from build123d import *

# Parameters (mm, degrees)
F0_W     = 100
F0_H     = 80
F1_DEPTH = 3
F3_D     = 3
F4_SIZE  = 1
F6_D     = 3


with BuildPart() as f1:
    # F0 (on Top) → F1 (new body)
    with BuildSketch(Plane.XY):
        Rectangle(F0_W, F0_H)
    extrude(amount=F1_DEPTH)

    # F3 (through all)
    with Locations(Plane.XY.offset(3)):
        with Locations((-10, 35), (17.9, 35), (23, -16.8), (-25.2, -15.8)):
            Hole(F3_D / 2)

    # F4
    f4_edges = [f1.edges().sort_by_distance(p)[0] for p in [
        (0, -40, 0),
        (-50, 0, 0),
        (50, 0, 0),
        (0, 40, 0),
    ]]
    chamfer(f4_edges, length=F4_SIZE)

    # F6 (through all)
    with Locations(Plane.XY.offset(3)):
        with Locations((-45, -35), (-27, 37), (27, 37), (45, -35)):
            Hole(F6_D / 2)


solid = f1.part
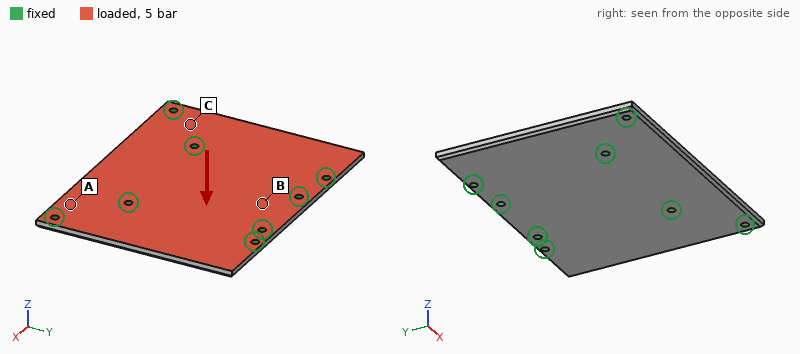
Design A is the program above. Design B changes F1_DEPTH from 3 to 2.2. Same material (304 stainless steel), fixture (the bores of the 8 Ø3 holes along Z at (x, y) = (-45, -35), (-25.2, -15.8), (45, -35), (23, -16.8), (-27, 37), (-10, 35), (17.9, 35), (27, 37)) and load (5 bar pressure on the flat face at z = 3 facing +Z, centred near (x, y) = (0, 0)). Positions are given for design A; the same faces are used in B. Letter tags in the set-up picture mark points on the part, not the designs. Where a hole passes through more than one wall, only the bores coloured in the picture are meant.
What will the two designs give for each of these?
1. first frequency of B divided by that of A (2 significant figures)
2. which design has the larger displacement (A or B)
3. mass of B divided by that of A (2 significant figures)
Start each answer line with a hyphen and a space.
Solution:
- 0.75
- B
- 0.73
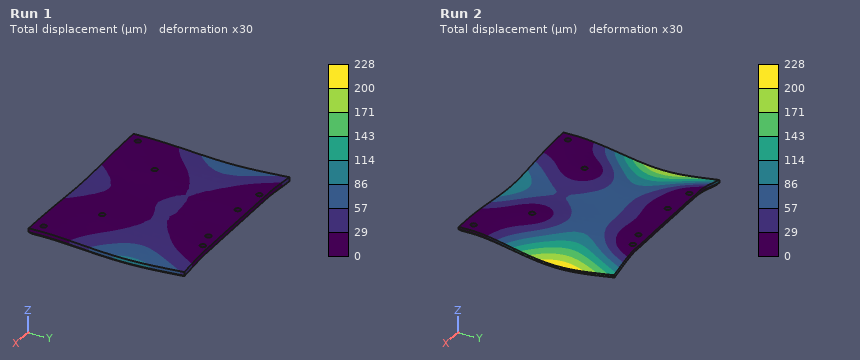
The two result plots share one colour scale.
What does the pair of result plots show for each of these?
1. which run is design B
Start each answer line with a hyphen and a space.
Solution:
- Run 2
